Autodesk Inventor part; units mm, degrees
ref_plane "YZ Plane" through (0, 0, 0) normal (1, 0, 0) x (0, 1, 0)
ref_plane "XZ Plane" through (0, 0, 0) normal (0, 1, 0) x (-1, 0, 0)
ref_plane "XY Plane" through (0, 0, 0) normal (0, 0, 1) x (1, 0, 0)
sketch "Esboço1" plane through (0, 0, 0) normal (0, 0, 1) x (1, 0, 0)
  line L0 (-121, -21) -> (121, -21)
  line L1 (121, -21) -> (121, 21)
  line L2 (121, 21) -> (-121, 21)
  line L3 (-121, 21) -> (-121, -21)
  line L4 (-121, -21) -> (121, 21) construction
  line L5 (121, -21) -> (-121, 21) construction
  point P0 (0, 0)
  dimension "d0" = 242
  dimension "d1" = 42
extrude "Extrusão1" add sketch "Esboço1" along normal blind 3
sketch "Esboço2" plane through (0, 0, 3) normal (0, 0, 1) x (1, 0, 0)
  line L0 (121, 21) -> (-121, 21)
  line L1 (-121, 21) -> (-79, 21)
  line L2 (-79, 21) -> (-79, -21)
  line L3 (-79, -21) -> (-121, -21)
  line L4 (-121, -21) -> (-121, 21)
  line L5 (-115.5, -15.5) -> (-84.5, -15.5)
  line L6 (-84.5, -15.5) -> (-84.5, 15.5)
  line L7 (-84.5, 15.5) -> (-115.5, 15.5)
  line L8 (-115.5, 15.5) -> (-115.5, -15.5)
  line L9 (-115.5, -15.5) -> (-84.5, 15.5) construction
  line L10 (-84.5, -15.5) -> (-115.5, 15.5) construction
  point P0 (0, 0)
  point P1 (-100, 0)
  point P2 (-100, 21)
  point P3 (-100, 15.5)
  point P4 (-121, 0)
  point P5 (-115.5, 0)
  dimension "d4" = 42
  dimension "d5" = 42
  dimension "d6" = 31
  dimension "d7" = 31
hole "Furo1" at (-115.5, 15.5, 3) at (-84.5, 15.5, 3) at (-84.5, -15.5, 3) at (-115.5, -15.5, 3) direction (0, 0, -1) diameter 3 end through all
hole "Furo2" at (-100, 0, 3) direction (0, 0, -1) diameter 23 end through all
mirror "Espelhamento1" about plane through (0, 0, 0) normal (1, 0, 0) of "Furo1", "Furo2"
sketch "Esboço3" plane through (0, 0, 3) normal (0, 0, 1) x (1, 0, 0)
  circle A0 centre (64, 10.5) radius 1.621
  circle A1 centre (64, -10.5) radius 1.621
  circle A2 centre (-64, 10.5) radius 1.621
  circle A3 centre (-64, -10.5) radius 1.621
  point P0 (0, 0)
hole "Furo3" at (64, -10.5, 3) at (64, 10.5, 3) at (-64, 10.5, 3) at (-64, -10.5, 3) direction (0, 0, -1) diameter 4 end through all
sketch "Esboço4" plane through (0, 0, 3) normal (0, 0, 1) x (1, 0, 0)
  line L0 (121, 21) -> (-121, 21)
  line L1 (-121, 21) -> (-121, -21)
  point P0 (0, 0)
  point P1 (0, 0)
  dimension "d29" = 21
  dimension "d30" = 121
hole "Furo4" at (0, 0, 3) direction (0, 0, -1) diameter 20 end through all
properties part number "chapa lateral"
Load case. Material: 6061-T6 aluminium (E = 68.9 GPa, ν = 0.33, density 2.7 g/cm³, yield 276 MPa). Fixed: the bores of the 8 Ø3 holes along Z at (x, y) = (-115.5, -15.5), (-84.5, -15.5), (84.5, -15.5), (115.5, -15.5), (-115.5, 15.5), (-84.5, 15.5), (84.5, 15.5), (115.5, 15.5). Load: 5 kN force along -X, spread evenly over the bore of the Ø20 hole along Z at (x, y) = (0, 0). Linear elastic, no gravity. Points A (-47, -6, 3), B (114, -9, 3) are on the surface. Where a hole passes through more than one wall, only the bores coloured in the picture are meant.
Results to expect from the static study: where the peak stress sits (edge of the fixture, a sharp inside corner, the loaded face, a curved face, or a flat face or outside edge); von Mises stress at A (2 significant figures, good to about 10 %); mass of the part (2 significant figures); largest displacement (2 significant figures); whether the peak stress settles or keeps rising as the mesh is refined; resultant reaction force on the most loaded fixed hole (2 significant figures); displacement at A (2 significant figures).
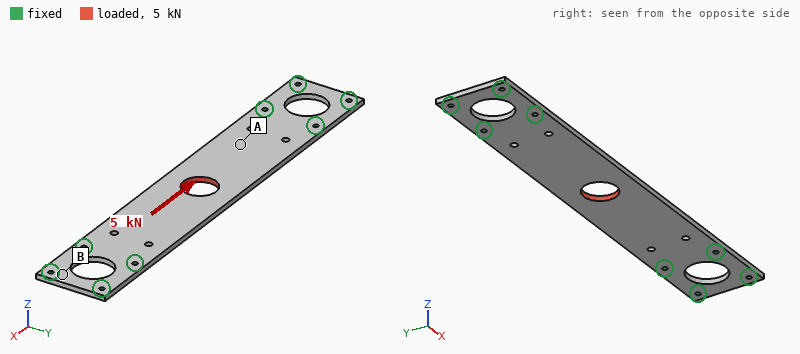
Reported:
edge of the fixture
20 MPa
72 g
28 µm
keeps rising
1.2 kN
14 µm
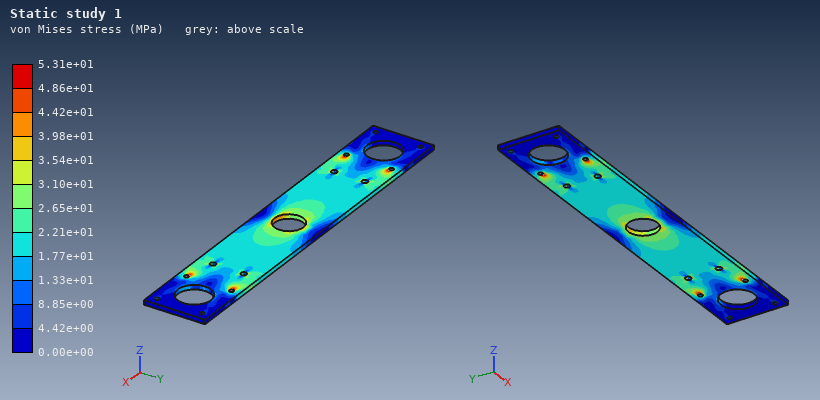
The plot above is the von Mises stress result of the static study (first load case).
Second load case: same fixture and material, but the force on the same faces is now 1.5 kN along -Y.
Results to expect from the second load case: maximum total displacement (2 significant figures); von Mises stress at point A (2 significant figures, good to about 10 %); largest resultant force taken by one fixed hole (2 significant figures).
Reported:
55 µm
14 MPa
980 N
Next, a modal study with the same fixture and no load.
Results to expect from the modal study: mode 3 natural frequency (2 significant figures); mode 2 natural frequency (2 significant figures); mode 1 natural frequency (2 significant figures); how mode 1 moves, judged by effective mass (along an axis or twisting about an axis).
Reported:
1500 Hz
1500 Hz
530 Hz
along Z
